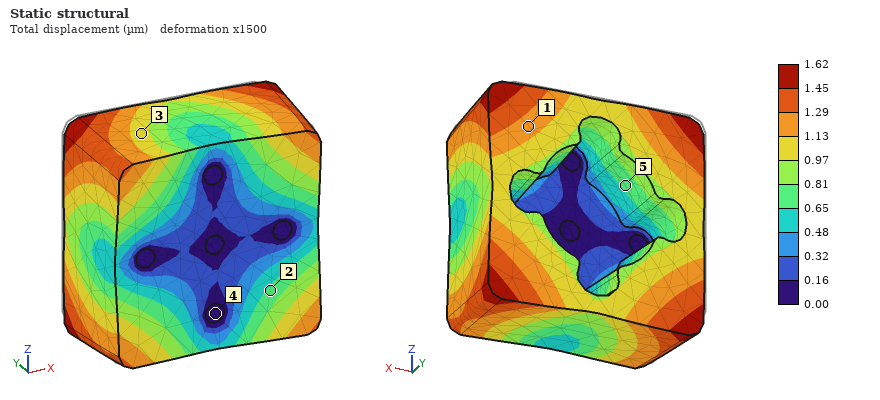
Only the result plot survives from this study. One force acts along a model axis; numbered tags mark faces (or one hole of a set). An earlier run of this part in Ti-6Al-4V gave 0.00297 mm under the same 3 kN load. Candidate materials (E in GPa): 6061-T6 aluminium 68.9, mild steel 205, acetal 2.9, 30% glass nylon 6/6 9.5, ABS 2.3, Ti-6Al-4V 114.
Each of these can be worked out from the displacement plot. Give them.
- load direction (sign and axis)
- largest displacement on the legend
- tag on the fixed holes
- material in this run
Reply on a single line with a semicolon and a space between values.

-Y; 1.62 µm; 4; mild steel
